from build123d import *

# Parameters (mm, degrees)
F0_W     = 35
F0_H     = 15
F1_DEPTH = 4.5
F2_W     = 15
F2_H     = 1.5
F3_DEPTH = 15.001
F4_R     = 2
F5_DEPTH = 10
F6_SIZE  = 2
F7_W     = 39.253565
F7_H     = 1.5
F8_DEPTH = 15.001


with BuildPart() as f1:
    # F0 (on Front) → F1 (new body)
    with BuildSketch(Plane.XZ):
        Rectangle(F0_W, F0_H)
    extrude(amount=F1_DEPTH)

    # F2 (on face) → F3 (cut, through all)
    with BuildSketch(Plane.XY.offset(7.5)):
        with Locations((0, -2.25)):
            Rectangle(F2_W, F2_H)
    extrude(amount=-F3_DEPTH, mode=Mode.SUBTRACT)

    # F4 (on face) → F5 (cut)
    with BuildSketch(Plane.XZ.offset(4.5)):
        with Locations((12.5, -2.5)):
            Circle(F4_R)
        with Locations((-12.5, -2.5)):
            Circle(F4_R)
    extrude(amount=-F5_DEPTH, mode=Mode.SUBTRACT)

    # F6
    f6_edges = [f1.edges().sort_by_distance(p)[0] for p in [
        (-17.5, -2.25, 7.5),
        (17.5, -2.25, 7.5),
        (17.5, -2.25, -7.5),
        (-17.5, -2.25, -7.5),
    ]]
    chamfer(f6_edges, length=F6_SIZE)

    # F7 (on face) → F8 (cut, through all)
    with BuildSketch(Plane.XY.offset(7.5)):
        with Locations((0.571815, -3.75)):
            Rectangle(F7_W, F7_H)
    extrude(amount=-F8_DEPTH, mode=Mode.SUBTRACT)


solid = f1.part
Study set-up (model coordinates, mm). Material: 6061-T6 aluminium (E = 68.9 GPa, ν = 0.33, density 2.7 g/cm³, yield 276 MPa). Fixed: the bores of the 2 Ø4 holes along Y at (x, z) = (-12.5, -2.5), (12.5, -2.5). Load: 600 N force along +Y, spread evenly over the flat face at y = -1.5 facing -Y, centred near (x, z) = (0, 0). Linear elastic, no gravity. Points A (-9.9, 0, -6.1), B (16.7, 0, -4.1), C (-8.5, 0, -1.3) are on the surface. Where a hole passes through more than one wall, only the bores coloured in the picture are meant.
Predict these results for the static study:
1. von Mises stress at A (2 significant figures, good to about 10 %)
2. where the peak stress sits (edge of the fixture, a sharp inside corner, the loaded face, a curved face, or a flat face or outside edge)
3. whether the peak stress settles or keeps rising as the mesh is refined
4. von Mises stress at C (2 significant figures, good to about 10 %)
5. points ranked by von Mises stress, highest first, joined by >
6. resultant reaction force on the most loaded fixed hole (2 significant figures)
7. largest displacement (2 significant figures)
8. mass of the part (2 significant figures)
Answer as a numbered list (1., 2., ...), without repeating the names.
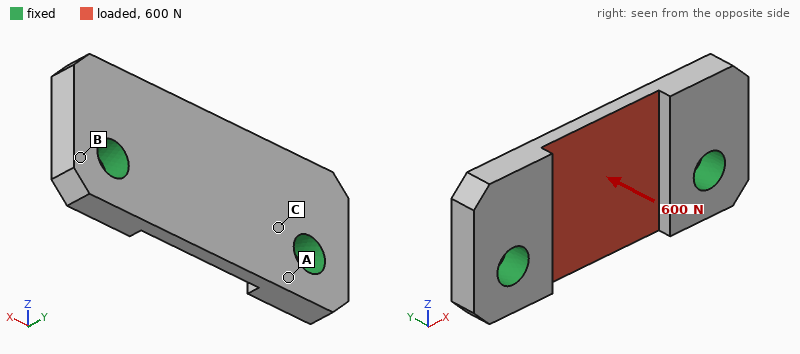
1. 37 MPa
2. edge of the fixture
3. keeps rising
4. 73 MPa
5. C > A > B
6. 350 N
7. 61 µm
8. 3.1 g
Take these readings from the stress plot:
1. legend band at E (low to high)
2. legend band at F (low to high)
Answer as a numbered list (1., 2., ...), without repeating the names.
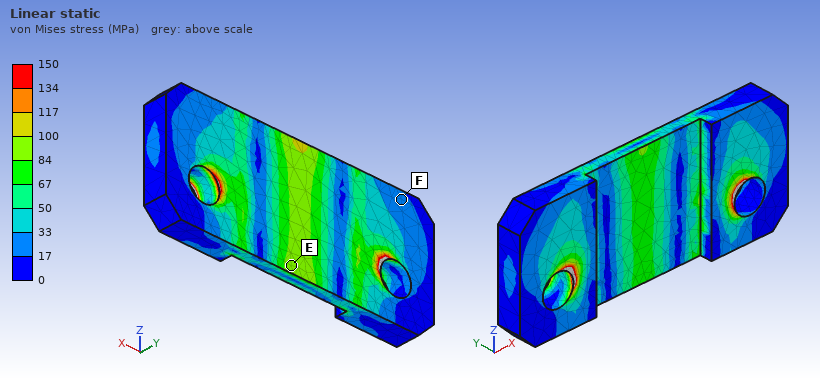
1. 84 to 100 MPa
2. 17 to 33 MPa
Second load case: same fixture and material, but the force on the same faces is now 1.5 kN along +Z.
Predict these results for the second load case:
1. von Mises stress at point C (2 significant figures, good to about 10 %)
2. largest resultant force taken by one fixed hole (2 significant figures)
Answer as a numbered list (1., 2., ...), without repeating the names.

1. 52 MPa
2. 780 N
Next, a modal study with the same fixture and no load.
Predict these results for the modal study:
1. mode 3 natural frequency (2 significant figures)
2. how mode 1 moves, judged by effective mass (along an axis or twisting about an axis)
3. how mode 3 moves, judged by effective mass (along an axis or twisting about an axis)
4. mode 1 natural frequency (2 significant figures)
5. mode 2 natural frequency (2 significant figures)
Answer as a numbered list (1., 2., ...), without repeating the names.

1. 29 kHz
2. along Y
3. twisting about Z
4. 20 kHz
5. 26 kHz
